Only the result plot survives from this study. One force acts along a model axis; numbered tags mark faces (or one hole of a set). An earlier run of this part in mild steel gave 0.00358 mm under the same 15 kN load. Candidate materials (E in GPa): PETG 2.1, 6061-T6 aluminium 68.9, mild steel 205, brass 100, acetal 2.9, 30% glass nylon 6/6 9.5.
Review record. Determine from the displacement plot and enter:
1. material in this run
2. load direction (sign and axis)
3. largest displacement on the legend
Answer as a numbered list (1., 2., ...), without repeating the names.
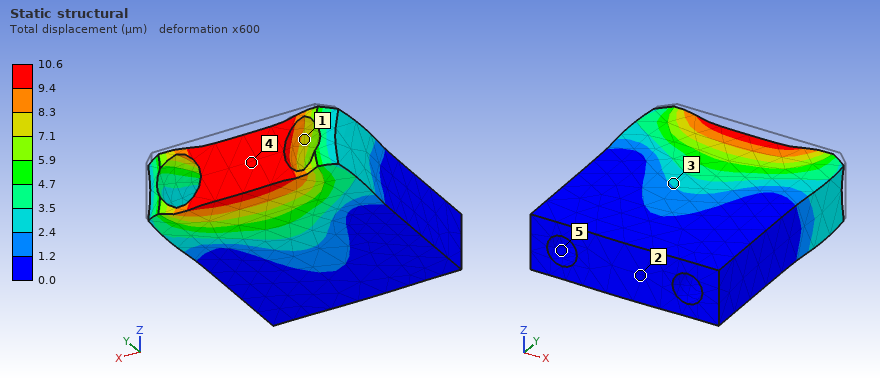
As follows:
1. 6061-T6 aluminium
2. -Y
3. 10.6 µm
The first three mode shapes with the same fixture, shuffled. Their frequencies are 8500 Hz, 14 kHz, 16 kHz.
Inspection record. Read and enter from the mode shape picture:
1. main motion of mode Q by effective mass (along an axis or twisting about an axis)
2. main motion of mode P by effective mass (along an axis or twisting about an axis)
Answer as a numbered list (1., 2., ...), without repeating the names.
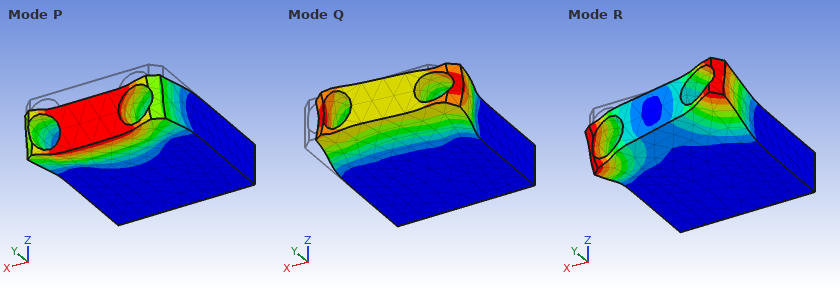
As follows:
1. along X
2. along Z
